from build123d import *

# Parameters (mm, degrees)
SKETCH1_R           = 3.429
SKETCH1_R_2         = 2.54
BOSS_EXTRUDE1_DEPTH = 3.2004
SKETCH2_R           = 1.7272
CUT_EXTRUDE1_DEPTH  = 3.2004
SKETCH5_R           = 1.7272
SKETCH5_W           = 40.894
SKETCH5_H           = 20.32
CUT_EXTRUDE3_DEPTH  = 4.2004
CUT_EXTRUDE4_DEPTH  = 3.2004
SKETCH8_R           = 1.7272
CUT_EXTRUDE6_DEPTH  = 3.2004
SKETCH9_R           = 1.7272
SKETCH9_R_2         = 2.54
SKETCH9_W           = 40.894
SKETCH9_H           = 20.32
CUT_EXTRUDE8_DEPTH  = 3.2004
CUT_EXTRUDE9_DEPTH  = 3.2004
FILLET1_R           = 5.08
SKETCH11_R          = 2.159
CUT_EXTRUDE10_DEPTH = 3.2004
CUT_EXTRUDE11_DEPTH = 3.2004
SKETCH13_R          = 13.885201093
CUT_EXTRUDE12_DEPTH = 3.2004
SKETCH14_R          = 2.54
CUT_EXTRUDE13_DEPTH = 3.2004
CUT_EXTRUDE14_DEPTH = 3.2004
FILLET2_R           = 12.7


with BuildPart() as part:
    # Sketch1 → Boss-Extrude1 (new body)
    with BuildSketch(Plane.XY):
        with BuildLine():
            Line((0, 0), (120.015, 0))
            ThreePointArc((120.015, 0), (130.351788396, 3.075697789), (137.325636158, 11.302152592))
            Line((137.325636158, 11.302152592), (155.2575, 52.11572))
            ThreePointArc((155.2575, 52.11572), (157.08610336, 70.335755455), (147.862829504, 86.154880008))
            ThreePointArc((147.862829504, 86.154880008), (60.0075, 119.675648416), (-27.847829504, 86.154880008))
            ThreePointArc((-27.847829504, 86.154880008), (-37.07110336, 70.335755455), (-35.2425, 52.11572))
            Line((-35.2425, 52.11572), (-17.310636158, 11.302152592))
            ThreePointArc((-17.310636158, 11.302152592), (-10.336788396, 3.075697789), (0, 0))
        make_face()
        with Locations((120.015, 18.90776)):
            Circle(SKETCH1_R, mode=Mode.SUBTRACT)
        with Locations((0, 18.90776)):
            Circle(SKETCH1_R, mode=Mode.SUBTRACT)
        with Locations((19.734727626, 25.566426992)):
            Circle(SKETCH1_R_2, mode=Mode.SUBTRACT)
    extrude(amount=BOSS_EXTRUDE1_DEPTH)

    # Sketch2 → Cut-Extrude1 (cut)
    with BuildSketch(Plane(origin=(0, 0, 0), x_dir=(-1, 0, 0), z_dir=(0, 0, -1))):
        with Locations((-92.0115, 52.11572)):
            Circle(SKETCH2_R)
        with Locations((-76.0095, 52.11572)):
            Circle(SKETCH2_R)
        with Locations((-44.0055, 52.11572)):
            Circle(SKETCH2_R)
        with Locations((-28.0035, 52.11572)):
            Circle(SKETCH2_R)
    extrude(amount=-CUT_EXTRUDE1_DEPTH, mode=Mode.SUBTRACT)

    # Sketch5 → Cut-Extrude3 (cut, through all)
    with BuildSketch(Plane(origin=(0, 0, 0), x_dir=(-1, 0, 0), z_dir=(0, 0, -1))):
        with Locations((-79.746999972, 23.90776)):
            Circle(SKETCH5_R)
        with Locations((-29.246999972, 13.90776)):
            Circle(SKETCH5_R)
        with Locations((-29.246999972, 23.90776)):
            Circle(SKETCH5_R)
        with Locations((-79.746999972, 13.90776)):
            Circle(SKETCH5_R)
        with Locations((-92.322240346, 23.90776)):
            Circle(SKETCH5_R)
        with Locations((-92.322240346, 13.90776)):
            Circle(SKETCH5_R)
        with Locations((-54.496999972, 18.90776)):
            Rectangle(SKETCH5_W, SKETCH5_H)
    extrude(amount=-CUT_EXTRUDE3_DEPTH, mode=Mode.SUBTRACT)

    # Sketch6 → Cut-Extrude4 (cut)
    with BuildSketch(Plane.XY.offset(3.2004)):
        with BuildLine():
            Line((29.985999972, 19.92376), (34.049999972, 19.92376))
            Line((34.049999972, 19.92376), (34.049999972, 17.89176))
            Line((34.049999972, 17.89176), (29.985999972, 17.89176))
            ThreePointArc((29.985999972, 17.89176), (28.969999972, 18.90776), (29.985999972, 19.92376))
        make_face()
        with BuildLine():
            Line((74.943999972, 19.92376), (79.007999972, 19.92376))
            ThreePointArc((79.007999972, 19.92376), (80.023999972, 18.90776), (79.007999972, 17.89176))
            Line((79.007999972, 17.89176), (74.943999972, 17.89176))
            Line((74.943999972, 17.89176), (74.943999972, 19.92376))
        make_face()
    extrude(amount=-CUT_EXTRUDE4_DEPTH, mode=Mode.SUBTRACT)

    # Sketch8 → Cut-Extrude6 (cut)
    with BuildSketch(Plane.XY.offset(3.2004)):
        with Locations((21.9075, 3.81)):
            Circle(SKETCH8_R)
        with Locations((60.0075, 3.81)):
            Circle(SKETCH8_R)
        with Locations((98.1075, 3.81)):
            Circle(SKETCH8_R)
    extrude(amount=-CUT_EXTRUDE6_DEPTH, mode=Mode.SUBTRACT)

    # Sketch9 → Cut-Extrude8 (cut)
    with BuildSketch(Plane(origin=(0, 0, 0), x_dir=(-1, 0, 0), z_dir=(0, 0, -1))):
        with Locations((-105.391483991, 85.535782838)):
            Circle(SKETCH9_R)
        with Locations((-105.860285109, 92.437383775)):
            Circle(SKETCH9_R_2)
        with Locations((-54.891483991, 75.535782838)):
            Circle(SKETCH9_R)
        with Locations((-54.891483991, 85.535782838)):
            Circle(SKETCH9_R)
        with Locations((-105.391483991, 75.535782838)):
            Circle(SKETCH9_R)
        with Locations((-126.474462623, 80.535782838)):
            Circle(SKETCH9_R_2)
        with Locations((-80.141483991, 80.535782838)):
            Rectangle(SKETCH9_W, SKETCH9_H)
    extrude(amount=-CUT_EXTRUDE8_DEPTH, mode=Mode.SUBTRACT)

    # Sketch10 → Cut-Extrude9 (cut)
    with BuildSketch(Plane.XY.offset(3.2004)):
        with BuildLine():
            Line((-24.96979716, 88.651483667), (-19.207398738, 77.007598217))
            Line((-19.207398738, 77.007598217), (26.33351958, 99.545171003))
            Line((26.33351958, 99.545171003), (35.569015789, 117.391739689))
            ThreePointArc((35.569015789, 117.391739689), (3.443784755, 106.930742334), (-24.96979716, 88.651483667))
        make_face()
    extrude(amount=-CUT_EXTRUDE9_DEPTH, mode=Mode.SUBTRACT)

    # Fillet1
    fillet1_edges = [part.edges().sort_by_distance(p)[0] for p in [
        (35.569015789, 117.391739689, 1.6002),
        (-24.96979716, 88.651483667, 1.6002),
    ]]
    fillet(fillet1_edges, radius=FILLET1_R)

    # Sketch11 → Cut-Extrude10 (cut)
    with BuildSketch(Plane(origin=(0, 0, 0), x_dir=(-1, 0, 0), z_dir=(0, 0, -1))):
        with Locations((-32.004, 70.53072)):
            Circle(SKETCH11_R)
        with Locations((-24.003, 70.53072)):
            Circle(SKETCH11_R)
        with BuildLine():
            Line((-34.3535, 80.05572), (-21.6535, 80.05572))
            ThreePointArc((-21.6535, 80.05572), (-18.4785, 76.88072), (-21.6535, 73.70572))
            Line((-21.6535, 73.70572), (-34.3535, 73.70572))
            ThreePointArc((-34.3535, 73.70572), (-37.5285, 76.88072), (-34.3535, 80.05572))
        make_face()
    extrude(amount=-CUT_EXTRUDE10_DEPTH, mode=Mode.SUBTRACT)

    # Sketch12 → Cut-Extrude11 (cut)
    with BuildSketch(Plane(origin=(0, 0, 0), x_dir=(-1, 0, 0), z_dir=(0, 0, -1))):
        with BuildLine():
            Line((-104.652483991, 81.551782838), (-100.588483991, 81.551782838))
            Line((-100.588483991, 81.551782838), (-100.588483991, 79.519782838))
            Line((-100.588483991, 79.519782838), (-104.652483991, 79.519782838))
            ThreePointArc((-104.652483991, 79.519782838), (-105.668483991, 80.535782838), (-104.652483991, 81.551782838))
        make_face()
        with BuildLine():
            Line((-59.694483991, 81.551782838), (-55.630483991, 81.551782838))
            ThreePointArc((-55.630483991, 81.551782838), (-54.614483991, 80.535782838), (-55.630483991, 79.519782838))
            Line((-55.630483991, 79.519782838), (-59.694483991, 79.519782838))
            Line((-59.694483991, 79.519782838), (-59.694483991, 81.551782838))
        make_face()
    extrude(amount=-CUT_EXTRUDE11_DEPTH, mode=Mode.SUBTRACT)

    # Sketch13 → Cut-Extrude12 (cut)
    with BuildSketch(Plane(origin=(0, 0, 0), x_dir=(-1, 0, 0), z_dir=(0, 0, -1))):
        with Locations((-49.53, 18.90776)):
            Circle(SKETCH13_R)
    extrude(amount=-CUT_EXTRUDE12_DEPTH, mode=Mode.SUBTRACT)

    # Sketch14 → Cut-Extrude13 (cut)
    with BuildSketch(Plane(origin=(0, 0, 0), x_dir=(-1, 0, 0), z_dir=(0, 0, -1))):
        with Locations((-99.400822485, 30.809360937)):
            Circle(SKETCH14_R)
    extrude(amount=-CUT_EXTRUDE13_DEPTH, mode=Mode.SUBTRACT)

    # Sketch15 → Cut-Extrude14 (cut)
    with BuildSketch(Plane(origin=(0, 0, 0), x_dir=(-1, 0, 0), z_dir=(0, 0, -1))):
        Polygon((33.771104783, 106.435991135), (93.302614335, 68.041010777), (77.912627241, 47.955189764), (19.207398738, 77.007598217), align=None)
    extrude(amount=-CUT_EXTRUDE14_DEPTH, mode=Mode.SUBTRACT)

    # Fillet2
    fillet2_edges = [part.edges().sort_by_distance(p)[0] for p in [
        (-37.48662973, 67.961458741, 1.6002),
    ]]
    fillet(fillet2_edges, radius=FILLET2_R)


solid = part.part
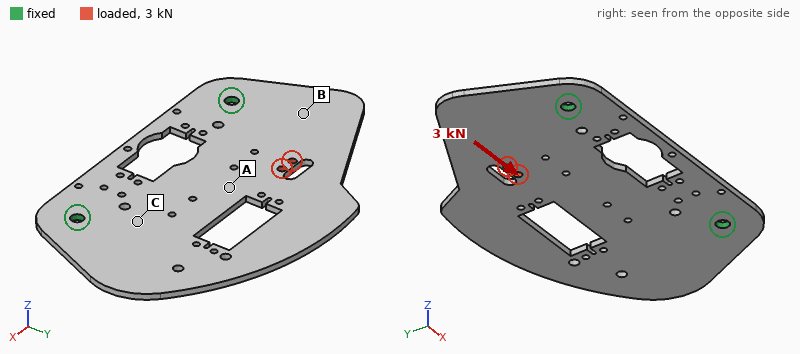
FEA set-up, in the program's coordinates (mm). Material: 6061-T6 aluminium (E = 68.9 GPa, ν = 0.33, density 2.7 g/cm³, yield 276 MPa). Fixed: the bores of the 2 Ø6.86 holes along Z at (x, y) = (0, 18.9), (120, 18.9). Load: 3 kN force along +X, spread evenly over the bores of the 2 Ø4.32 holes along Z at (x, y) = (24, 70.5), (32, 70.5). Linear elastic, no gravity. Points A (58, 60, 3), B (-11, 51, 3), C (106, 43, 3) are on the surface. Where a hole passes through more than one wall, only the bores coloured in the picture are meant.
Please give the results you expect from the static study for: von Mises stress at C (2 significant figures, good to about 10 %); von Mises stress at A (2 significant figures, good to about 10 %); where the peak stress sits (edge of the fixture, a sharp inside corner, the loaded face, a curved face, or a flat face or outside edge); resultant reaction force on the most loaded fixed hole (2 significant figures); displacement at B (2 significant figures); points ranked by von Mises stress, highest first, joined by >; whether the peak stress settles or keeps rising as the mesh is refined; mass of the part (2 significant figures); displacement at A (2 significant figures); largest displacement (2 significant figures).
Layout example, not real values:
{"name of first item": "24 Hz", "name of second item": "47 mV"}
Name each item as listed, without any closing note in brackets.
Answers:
{"von Mises stress at C": "11 MPa", "von Mises stress at A": "20 MPa", "where the peak stress sits": "a sharp inside corner", "resultant reaction force on the most loaded fixed hole": "2.0 kN", "displacement at B": "23 µm", "points ranked by von Mises stress, highest first, joined by >": "A > C > B", "whether the peak stress settles or keeps rising as the mesh is refined": "keeps rising", "mass of the part": "140 g", "displacement at A": "22 µm", "largest displacement": "43 µm"}
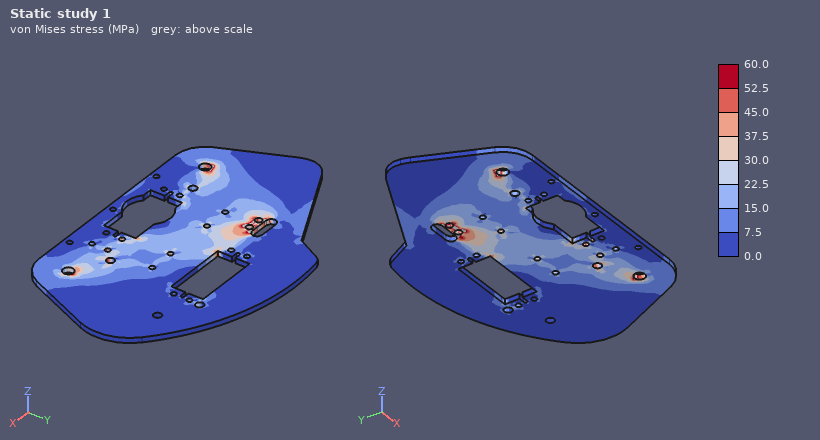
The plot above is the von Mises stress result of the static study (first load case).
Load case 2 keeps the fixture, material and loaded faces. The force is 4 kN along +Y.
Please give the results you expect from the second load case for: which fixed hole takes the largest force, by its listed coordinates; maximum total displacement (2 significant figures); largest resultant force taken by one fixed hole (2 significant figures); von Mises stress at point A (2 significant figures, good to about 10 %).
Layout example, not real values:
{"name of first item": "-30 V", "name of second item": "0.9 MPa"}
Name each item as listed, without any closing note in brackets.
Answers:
{"which fixed hole takes the largest force, by its listed coordinates": "(0, 18.9)", "maximum total displacement": "46 µm", "largest resultant force taken by one fixed hole": "3.2 kN", "von Mises stress at point A": "12 MPa"}
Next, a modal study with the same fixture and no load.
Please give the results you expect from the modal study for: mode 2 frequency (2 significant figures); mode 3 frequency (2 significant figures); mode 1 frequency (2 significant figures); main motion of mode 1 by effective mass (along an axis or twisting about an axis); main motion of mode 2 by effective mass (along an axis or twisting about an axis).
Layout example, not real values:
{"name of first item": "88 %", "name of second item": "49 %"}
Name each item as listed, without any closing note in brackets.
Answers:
{"mode 2 frequency": "590 Hz", "mode 3 frequency": "950 Hz", "mode 1 frequency": "280 Hz", "main motion of mode 1 by effective mass": "along Z", "main motion of mode 2 by effective mass": "twisting about Y"}
